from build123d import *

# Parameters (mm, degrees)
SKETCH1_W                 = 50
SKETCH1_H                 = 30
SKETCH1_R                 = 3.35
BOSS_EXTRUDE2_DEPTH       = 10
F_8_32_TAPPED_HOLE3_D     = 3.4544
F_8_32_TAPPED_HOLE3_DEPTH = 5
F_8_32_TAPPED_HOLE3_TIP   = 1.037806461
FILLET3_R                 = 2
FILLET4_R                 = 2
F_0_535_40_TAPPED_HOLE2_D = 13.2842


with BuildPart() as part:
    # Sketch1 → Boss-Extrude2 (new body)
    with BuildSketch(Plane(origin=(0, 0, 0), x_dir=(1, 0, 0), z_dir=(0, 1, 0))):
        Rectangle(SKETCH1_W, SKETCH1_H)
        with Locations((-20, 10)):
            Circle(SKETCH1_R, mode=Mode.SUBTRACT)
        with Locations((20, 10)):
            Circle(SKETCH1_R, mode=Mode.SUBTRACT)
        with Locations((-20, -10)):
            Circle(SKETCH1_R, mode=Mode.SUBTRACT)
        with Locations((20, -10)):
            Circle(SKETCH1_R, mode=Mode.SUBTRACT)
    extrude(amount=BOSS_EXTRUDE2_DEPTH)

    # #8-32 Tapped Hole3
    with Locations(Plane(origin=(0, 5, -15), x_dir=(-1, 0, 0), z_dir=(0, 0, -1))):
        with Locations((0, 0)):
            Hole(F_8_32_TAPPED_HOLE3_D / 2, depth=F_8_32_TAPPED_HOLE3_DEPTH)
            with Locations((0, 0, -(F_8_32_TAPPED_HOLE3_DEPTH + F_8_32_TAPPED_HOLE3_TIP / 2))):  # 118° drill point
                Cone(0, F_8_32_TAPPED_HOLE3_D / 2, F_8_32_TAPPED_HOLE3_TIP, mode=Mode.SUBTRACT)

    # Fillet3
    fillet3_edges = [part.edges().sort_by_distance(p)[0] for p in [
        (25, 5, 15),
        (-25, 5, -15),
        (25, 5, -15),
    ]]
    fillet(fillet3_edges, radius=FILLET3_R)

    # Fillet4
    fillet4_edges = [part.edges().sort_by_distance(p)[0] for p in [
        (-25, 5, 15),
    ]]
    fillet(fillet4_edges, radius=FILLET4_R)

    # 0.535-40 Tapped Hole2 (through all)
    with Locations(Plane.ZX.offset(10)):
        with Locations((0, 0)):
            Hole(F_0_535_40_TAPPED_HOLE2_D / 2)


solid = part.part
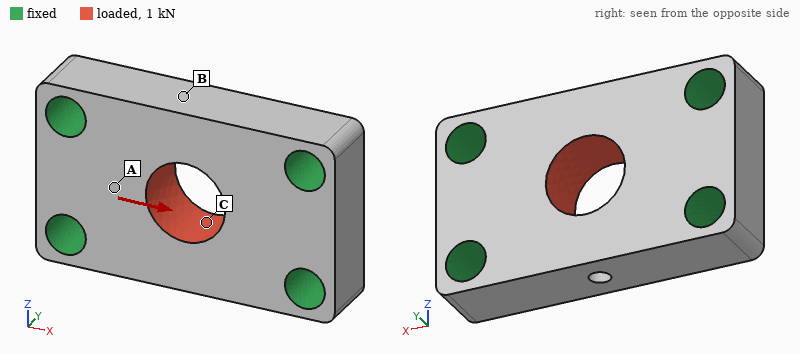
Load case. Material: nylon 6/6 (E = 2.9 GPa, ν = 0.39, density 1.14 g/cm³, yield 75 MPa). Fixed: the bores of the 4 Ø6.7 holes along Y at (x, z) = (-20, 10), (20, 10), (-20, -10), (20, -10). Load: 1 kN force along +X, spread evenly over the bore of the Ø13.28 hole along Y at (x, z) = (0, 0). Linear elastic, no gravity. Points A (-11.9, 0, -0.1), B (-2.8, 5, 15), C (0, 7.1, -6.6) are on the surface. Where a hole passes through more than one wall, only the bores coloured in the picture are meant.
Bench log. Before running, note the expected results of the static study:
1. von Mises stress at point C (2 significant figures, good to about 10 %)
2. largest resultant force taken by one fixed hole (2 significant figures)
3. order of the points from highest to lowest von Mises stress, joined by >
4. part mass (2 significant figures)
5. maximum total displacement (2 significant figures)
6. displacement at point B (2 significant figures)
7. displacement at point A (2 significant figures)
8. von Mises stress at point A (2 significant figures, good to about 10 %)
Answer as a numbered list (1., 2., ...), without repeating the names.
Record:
1. 4.2 MPa
2. 260 N
3. C > A > B
4. 14 g
5. 13 µm
6. 4.2 µm
7. 7.1 µm
8. 1.7 MPa
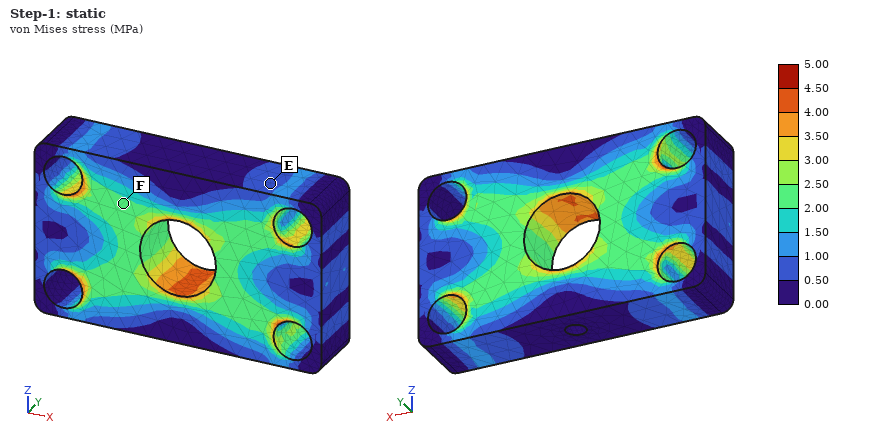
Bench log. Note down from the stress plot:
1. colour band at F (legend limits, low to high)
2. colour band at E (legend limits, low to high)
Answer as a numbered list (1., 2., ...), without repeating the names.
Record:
1. 2.00 to 2.50 MPa
2. 0.50 to 1.00 MPa
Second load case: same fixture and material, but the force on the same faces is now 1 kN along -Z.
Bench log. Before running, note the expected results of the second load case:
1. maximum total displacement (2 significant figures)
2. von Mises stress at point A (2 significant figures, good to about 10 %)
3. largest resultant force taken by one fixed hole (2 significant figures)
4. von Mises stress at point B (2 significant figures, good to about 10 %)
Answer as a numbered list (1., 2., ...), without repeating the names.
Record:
1. 36 µm
2. 4.4 MPa
3. 320 N
4. 3.5 MPa
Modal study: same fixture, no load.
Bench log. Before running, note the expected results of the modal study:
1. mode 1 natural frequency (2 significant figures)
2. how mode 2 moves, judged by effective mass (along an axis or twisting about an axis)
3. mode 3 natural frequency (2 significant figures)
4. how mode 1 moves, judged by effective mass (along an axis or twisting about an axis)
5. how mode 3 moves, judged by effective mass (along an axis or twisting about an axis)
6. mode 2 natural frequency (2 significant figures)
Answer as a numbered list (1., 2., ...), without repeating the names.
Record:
1. 9300 Hz
2. twisting about X
3. 13 kHz
4. along Y
5. along Z
6. 11 kHz
